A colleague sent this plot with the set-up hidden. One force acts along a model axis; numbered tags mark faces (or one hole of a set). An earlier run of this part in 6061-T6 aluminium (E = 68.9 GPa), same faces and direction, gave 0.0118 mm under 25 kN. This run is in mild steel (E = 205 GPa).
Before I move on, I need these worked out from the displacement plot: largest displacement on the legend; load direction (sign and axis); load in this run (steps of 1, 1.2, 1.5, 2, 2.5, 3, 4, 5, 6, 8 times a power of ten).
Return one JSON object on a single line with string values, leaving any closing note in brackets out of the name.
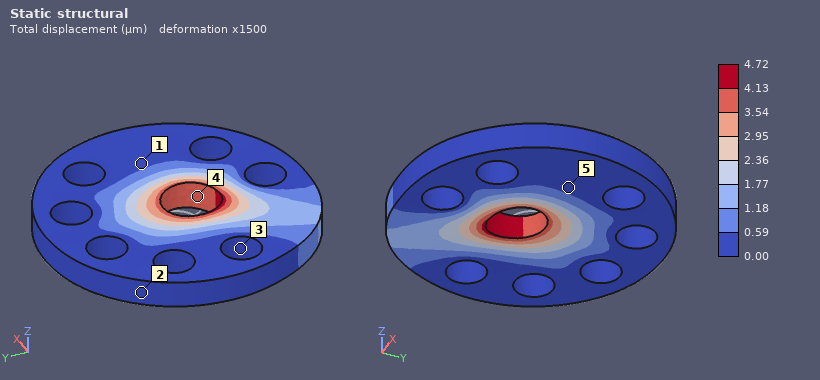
{"largest displacement on the legend": "4.72 µm", "load direction": "-Y", "load in this run": "30 kN"}
